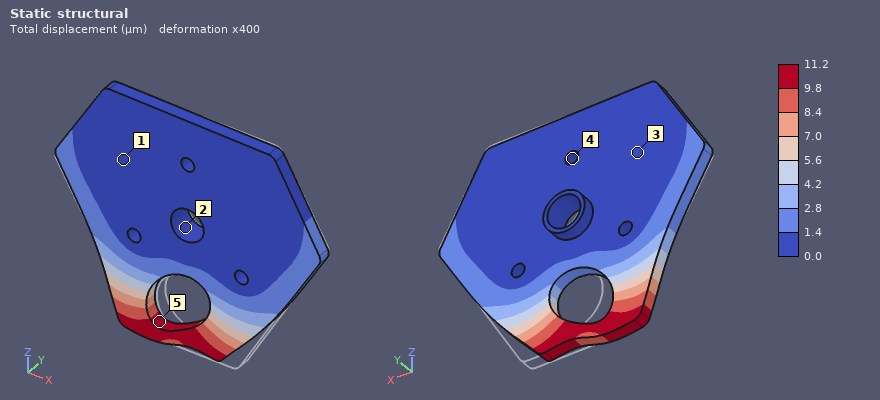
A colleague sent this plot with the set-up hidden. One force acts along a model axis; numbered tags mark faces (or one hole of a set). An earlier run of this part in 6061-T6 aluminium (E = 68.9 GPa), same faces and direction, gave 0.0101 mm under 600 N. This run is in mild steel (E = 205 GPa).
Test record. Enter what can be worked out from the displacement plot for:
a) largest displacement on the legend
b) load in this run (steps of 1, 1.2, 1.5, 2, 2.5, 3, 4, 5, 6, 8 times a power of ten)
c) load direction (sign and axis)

11.2 µm
2 kN
-X
